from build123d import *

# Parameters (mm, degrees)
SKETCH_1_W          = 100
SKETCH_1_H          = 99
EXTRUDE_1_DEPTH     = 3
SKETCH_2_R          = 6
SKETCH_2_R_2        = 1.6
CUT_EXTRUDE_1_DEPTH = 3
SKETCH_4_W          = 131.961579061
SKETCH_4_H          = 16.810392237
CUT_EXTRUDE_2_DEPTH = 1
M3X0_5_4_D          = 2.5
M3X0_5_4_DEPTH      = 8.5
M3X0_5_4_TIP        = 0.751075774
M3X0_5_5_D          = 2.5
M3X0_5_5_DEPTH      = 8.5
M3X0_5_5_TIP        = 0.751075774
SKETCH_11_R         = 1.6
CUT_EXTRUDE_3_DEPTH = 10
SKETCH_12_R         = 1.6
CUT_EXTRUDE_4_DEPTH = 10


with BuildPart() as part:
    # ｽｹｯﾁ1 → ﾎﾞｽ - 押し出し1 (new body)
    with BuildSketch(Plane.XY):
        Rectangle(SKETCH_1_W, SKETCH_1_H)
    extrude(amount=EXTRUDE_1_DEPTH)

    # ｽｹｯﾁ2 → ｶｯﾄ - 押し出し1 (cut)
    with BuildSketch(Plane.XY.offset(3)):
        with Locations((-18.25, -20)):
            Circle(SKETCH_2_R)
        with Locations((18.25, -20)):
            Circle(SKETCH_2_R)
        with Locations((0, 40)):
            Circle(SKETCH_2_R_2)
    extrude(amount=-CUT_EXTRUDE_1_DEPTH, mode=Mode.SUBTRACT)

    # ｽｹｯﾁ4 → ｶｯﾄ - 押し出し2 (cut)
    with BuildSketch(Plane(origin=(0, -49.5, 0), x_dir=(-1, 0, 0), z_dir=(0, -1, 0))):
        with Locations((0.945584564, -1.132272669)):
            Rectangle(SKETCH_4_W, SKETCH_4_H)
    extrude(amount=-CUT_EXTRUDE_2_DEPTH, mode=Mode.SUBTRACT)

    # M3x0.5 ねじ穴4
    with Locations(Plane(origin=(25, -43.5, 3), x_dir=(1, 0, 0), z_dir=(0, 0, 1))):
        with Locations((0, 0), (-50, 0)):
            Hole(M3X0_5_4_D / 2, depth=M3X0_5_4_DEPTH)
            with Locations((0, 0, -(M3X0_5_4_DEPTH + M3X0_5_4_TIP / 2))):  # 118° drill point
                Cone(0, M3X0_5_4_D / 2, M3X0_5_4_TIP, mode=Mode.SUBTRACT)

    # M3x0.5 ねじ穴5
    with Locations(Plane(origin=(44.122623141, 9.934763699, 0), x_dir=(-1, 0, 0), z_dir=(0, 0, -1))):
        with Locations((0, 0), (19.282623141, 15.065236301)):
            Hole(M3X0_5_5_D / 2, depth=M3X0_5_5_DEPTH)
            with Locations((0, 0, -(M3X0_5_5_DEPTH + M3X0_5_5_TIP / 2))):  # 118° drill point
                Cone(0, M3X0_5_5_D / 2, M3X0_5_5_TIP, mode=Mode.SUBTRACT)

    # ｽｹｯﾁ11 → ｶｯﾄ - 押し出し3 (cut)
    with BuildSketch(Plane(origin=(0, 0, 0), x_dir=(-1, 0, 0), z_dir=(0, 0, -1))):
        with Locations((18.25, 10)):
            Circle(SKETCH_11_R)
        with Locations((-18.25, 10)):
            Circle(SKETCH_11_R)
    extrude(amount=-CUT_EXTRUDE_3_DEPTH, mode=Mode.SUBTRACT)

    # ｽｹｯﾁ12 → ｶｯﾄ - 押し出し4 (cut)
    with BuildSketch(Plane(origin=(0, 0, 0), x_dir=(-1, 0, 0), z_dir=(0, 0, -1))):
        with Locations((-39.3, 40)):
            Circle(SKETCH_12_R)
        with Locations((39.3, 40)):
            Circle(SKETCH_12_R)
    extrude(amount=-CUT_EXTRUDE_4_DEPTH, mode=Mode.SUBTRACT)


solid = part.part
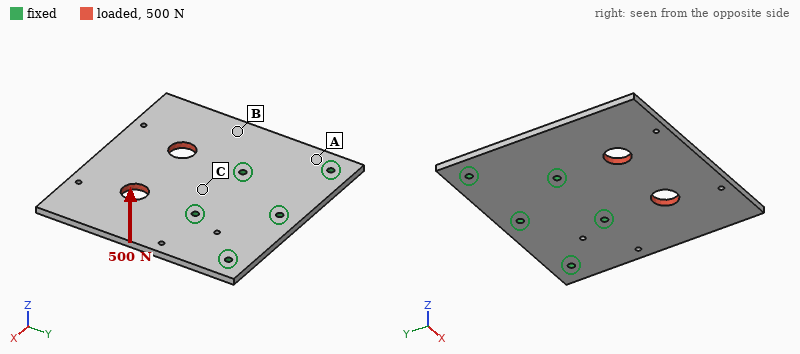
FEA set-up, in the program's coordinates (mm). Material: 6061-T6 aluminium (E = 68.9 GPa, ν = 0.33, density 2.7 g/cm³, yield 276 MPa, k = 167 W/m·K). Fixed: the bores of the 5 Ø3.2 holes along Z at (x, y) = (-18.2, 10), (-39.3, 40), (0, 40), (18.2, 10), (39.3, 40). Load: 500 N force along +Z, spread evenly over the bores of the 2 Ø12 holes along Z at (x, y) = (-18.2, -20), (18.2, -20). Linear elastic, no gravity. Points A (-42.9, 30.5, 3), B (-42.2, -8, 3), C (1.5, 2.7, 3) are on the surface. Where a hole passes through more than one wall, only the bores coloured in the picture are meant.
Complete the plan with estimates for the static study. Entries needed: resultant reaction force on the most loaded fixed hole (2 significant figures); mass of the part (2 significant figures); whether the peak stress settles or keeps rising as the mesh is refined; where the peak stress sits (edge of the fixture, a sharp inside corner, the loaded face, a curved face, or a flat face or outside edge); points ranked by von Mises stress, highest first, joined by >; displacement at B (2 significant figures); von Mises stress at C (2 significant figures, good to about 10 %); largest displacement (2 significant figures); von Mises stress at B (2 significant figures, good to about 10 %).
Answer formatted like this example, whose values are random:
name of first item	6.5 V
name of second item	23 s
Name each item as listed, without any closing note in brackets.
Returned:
resultant reaction force on the most loaded fixed hole	370 N
mass of the part	77 g
whether the peak stress settles or keeps rising as the mesh is refined	keeps rising
where the peak stress sits	edge of the fixture
points ranked by von Mises stress, highest first, joined by >	C > B > A
displacement at B	0.18 mm
von Mises stress at C	68 MPa
largest displacement	0.88 mm
von Mises stress at B	38 MPa
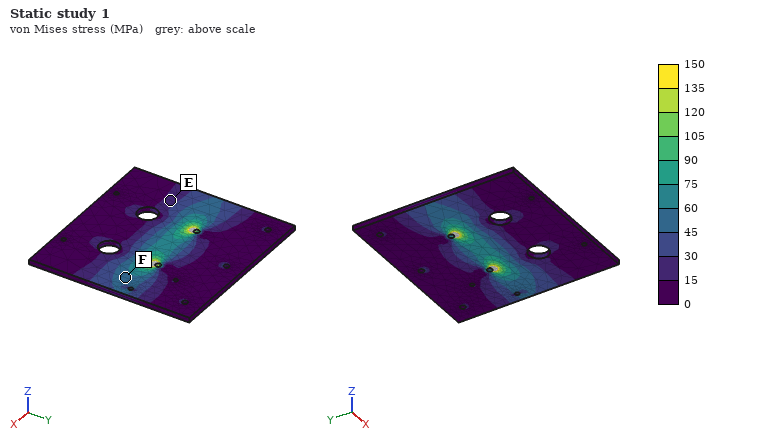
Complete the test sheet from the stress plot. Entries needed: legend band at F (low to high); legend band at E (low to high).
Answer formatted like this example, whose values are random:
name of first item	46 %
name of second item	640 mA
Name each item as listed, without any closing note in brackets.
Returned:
legend band at F	45 to 60 MPa
legend band at E	15 to 30 MPa
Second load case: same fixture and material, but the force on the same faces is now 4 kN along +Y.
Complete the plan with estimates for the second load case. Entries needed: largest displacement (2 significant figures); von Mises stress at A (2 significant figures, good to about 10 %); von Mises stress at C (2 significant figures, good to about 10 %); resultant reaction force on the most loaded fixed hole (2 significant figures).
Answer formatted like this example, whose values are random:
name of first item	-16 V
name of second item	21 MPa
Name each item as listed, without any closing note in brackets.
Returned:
largest displacement	14 µm
von Mises stress at A	8.9 MPa
von Mises stress at C	12 MPa
resultant reaction force on the most loaded fixed hole	1.3 kN
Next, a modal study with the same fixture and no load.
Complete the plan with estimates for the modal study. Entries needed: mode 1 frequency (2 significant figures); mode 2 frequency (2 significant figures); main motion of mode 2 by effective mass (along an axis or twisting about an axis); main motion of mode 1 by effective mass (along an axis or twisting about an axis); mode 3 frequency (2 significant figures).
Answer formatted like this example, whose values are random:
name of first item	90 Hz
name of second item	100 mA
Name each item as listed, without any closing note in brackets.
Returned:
mode 1 frequency	660 Hz
mode 2 frequency	970 Hz
main motion of mode 2 by effective mass	twisting about Y
main motion of mode 1 by effective mass	along Z
mode 3 frequency	2000 Hz
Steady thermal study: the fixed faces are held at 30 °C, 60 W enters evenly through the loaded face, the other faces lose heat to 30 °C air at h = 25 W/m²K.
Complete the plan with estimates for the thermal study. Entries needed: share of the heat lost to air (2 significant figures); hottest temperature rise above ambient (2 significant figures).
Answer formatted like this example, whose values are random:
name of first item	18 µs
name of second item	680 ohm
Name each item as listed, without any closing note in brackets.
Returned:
share of the heat lost to air	18 %
hottest temperature rise above ambient	51 K
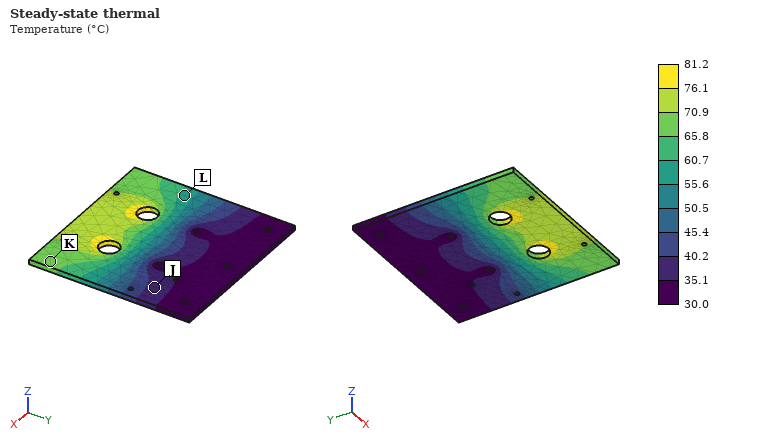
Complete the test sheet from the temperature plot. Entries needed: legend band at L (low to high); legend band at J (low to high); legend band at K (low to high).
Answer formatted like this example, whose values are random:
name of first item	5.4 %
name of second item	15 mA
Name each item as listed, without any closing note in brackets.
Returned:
legend band at L	55.6 to 60.7 °C
legend band at J	35.1 to 40.2 °C
legend band at K	65.8 to 70.9 °C
